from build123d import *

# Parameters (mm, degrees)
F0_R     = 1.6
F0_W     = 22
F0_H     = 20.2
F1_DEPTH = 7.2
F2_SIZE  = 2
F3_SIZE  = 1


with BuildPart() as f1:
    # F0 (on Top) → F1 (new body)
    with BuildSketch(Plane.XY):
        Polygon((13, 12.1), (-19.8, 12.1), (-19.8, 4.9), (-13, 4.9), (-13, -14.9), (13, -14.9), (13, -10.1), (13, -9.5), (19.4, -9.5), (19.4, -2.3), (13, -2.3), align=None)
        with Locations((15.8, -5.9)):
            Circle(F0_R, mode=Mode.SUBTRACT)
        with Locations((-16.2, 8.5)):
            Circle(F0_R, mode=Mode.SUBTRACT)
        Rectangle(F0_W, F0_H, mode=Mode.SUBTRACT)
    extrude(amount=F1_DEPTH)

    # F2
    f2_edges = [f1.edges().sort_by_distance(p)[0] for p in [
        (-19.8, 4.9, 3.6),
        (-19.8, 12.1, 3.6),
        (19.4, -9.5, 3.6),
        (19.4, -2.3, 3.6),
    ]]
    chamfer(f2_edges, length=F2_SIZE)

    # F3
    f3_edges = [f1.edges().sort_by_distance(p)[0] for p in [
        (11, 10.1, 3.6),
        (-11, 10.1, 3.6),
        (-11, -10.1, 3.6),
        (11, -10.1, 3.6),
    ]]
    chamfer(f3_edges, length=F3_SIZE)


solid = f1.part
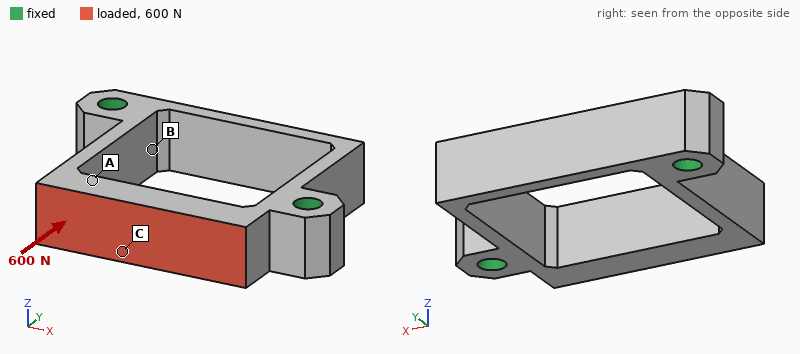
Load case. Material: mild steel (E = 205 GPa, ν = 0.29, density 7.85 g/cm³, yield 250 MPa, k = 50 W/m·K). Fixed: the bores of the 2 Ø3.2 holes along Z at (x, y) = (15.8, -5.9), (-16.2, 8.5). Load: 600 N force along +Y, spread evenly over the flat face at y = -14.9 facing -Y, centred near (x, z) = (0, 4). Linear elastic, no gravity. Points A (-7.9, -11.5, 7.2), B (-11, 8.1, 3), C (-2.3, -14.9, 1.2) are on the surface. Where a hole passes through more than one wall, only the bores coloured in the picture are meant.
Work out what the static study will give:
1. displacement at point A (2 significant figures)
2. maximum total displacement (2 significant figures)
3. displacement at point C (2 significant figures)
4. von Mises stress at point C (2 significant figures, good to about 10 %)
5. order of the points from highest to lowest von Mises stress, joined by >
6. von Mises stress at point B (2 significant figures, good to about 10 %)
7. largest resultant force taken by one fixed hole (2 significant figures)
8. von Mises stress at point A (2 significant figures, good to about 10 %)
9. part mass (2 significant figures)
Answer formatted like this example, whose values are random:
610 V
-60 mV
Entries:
5.7 µm
7.8 µm
7.4 µm
44 MPa
C > A > B
6.6 MPa
310 N
16 MPa
19 g
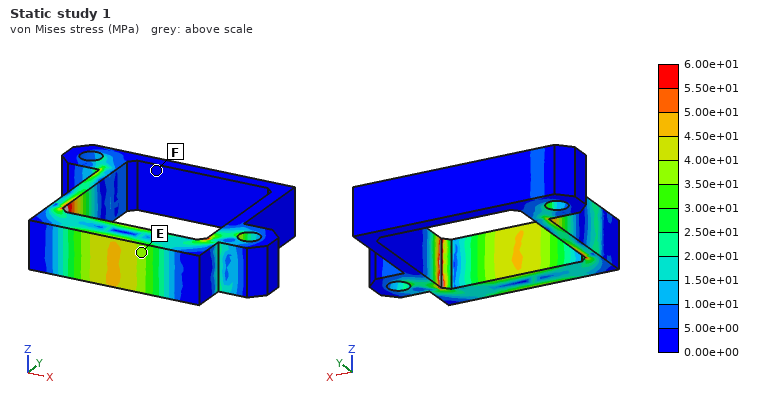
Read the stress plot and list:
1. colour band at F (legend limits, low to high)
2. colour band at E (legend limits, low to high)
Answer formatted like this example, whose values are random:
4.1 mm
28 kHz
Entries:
0.00e+00 to 5.00e+00 MPa
3.50e+01 to 4.00e+01 MPa
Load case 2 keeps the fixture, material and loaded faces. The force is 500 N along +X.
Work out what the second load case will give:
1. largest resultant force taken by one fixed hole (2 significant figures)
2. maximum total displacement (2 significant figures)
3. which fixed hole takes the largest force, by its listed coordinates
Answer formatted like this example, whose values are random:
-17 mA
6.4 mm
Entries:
500 N
5.4 µm
(15.8, -5.9)
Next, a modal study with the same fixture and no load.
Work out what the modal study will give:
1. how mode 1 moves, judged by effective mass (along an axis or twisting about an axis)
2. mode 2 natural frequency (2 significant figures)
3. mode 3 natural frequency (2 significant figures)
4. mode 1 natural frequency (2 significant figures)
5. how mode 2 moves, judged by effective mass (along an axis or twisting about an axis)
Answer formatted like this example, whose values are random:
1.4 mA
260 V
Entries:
along Z
14 kHz
15 kHz
8300 Hz
along Z
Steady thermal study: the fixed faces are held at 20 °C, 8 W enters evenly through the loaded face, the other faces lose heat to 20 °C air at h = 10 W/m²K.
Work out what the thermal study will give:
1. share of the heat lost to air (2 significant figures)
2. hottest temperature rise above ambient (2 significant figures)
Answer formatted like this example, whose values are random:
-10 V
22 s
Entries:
4.0 %
56 K
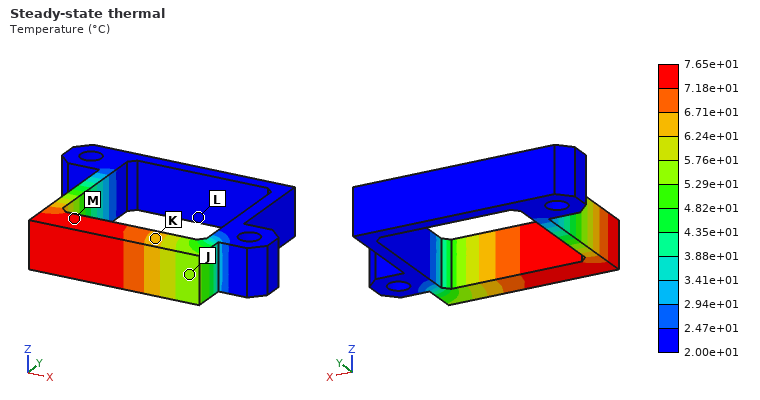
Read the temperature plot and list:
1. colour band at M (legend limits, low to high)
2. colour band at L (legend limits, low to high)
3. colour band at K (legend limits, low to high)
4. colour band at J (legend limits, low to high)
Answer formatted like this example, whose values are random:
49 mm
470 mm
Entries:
7.18e+01 to 7.65e+01 °C
2.00e+01 to 2.47e+01 °C
6.24e+01 to 6.71e+01 °C
5.29e+01 to 5.76e+01 °C
